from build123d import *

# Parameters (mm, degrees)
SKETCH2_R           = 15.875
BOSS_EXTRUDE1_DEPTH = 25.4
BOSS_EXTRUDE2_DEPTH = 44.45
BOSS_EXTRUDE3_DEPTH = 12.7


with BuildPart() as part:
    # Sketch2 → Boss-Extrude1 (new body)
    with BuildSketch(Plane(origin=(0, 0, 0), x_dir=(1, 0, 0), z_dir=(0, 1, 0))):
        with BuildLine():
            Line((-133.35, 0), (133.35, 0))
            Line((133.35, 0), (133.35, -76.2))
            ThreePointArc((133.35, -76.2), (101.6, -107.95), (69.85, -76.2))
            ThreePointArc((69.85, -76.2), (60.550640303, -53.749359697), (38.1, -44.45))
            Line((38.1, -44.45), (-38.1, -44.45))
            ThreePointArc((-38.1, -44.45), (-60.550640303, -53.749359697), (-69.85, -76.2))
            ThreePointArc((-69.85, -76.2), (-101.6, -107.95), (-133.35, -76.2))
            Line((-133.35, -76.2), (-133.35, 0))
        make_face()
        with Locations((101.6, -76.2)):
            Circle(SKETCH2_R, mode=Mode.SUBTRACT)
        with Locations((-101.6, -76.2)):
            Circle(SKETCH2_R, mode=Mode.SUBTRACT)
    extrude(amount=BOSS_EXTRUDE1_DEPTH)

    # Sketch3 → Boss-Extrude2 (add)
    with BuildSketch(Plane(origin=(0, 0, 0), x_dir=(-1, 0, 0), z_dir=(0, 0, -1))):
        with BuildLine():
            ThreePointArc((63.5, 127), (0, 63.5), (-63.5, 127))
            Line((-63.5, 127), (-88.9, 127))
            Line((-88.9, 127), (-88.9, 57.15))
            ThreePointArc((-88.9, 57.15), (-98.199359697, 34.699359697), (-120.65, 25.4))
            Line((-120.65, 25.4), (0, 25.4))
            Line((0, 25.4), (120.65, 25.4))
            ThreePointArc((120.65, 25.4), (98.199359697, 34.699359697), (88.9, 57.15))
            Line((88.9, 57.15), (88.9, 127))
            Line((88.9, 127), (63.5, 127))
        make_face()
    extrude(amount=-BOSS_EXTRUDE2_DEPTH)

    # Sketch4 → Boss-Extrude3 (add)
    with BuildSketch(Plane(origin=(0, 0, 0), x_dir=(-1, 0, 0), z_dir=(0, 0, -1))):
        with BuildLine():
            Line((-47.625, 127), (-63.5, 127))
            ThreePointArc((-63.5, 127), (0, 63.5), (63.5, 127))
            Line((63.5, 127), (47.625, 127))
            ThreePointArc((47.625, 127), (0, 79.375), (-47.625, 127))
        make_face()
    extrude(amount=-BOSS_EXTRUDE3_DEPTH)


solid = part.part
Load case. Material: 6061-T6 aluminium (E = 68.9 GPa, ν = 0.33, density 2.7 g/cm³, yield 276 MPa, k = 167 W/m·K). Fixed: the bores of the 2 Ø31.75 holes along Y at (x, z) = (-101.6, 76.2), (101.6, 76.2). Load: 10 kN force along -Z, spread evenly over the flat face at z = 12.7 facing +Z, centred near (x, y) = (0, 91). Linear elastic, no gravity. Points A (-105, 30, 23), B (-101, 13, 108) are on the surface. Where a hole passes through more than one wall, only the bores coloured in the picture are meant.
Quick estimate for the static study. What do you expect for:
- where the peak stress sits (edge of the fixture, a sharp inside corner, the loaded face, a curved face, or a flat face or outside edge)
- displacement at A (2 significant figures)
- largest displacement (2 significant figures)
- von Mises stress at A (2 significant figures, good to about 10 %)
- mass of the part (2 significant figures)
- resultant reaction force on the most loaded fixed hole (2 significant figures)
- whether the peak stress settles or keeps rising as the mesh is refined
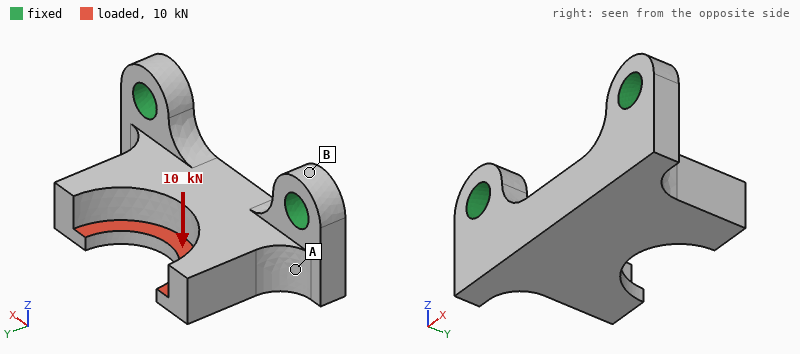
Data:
edge of the fixture
0.063 mm
0.34 mm
17 MPa
2.8 kg
5.8 kN
keeps rising
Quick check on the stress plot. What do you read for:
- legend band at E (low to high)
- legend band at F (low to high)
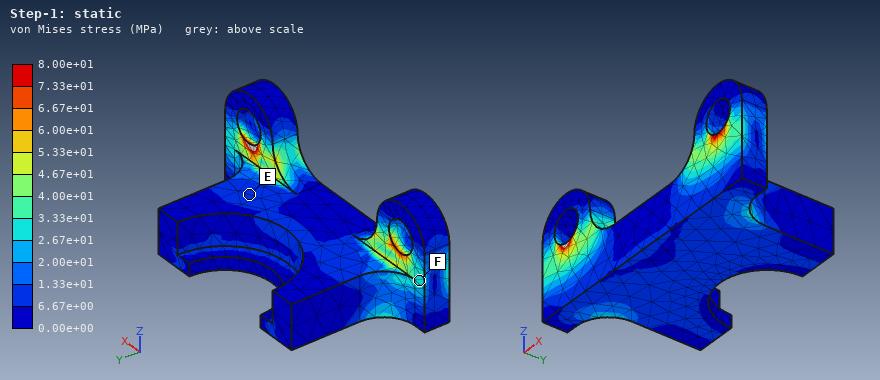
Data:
6.67e+00 to 1.33e+01 MPa
2.67e+01 to 3.33e+01 MPa
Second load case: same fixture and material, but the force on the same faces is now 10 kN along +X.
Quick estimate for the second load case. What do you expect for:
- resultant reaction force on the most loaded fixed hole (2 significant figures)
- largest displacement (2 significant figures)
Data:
6.6 kN
38 µm
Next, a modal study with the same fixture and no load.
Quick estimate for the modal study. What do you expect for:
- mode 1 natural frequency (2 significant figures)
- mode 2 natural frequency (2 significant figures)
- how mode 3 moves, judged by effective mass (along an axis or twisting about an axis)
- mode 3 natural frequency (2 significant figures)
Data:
1000 Hz
2300 Hz
along Y
3100 Hz
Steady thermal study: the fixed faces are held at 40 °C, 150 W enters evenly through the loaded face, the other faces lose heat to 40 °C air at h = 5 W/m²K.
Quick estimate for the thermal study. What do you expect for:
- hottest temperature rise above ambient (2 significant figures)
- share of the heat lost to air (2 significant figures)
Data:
28 K
3.9 %
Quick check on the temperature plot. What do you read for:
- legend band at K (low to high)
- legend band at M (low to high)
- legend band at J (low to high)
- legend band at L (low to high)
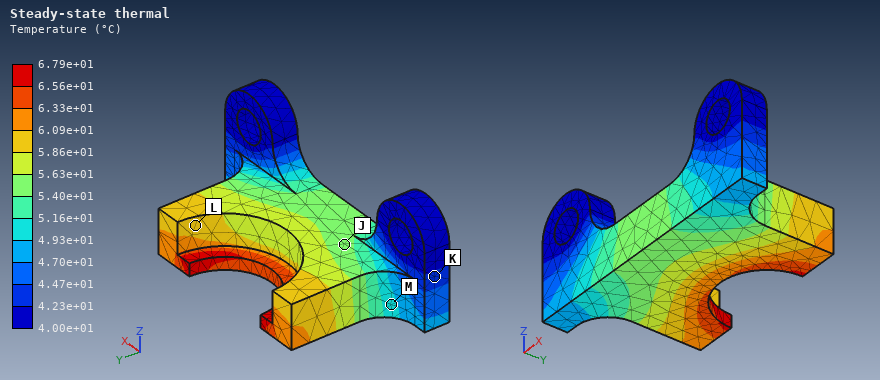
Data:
4.23e+01 to 4.47e+01 °C
4.93e+01 to 5.16e+01 °C
5.40e+01 to 5.63e+01 °C
5.86e+01 to 6.09e+01 °C
